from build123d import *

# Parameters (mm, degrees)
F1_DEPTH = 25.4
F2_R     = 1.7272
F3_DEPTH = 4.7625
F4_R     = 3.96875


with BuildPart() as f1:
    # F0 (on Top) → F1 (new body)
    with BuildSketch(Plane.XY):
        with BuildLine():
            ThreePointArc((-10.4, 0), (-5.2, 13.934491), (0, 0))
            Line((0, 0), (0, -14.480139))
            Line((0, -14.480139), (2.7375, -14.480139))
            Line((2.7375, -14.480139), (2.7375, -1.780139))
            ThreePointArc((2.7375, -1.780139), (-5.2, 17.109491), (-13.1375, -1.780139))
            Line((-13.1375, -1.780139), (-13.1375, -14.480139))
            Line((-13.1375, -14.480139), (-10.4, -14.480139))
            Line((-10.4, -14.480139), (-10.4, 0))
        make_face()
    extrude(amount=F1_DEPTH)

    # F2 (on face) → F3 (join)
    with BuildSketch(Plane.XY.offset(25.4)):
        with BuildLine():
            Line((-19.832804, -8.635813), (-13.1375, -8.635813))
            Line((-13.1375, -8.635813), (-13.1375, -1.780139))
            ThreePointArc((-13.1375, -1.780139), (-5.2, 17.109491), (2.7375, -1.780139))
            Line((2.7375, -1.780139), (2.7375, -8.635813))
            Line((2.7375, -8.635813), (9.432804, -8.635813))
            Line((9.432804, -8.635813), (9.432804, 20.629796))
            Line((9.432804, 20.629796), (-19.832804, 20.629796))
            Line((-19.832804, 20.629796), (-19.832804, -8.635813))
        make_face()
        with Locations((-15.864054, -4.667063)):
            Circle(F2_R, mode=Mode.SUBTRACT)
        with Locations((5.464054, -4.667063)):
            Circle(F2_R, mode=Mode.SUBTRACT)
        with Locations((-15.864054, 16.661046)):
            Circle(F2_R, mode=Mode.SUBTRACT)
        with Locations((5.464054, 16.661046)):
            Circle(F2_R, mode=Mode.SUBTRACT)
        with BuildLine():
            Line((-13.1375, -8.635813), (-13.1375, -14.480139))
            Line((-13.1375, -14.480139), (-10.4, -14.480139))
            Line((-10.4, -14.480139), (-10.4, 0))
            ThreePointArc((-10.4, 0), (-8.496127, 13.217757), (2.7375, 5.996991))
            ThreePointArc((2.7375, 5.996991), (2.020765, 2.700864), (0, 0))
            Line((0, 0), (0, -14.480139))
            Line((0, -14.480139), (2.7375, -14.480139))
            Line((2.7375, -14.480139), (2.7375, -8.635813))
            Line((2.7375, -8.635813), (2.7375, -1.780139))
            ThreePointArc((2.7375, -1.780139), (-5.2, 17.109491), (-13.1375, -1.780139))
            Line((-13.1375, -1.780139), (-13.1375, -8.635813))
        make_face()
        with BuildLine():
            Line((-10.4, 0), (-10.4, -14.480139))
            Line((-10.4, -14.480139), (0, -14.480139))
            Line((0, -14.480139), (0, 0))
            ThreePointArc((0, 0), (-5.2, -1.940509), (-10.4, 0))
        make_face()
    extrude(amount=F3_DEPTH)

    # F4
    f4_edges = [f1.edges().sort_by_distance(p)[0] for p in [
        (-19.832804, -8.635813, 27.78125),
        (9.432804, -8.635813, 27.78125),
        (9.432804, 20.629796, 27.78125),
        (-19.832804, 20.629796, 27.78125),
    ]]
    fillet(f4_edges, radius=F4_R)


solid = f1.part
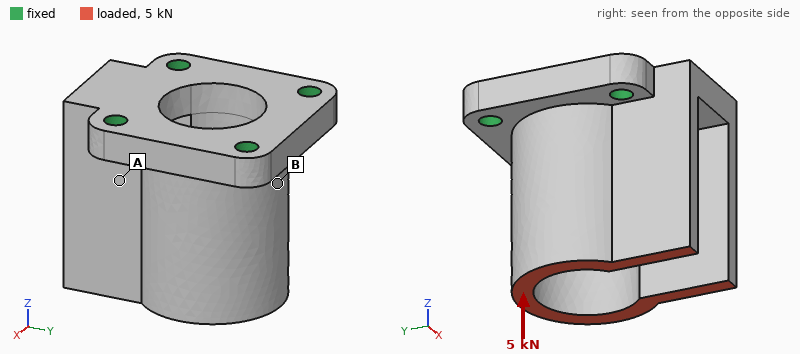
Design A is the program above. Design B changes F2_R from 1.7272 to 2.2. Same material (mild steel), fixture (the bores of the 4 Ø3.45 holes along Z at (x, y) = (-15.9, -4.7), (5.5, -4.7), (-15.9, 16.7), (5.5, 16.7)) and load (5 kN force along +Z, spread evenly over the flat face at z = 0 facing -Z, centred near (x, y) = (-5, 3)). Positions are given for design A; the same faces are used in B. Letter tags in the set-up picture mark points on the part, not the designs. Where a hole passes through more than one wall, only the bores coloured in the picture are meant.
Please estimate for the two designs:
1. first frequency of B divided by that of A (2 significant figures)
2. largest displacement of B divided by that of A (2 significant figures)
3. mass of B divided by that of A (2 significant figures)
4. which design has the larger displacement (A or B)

1.0
0.88
0.99
A
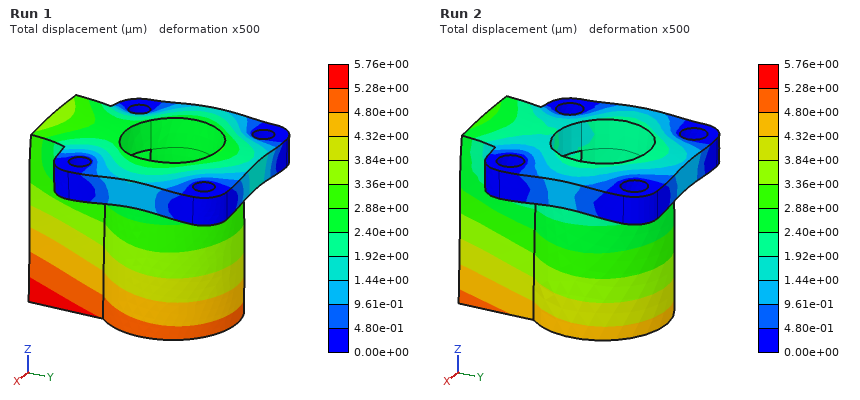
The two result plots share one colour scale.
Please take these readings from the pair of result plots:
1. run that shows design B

Run 2
